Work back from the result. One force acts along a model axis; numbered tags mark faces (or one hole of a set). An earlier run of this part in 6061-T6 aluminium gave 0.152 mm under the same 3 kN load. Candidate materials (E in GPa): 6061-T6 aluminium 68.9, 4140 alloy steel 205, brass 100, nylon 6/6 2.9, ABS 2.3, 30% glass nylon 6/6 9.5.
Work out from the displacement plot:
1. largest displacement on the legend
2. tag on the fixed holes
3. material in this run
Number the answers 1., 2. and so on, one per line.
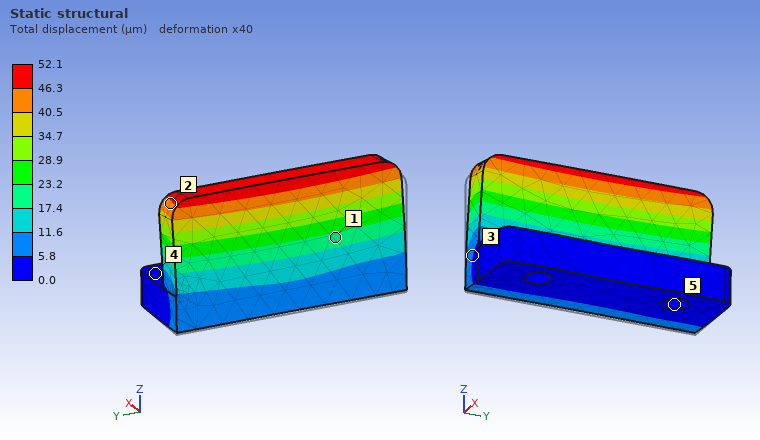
1. 52.1 µm
2. 5
3. 4140 alloy steel
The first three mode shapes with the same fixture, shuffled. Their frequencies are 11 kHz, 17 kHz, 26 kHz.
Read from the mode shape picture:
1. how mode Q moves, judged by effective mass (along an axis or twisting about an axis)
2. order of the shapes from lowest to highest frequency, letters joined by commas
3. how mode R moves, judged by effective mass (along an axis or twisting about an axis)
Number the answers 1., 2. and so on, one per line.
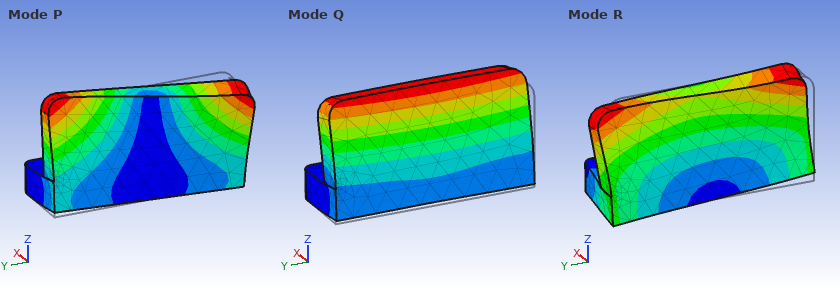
1. along X
2. Q, P, R
3. along Y
